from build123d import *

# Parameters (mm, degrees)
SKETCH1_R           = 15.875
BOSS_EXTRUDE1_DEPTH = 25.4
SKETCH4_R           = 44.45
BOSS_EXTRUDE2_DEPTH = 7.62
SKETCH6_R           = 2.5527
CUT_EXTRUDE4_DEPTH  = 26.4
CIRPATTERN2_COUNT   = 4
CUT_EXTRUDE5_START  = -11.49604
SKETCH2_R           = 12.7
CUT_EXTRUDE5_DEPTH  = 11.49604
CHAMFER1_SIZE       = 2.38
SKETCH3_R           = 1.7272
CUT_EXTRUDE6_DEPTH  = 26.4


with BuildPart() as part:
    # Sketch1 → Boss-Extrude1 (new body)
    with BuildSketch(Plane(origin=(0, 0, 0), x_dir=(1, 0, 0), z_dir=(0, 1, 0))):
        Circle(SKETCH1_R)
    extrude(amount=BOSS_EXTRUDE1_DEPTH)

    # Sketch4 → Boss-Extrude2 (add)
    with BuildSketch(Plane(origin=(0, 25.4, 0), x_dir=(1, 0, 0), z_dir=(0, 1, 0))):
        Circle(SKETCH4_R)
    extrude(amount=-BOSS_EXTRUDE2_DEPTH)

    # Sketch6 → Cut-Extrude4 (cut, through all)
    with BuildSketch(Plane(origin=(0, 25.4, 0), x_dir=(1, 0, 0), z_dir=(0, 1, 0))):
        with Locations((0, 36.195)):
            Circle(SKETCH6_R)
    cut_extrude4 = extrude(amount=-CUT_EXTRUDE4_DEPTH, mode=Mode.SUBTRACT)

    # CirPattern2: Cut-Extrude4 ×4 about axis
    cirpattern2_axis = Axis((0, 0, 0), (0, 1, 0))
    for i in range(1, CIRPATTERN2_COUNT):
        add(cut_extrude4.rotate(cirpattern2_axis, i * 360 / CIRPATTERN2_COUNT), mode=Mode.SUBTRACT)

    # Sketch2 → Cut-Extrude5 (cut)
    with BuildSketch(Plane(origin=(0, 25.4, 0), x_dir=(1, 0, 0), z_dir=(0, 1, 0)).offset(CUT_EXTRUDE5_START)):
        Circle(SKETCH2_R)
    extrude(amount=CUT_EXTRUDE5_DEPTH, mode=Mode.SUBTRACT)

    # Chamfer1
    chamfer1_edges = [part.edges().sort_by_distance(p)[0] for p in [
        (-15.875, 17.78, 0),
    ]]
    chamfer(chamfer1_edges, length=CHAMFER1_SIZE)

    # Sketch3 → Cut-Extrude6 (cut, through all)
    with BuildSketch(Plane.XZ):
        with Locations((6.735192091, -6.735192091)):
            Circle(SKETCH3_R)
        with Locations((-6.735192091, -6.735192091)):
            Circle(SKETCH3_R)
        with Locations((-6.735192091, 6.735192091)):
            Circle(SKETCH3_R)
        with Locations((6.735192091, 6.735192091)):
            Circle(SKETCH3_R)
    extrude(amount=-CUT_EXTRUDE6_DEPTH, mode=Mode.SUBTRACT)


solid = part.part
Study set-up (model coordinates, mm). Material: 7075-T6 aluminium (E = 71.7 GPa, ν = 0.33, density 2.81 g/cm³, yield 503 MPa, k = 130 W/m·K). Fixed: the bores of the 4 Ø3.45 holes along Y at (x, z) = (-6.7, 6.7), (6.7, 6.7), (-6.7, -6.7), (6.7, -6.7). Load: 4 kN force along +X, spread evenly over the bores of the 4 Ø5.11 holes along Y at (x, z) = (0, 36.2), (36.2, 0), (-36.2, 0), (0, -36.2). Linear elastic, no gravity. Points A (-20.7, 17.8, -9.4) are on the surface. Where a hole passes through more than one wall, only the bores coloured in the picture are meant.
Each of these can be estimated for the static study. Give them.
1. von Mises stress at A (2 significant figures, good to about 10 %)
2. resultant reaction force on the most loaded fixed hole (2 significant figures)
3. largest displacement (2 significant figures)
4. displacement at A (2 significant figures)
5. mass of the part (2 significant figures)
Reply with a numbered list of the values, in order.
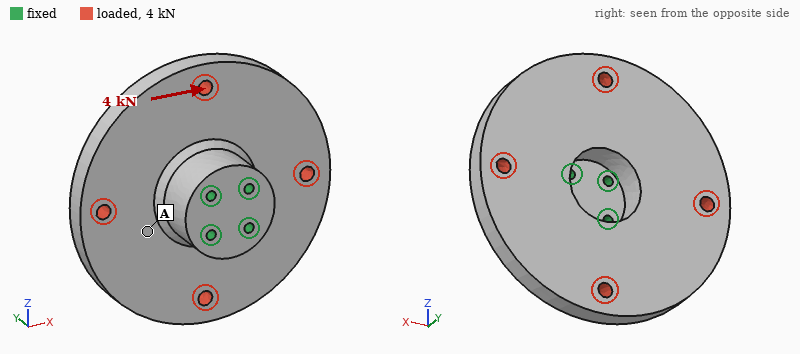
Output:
1. 7.7 MPa
2. 1.5 kN
3. 33 µm
4. 13 µm
5. 150 g
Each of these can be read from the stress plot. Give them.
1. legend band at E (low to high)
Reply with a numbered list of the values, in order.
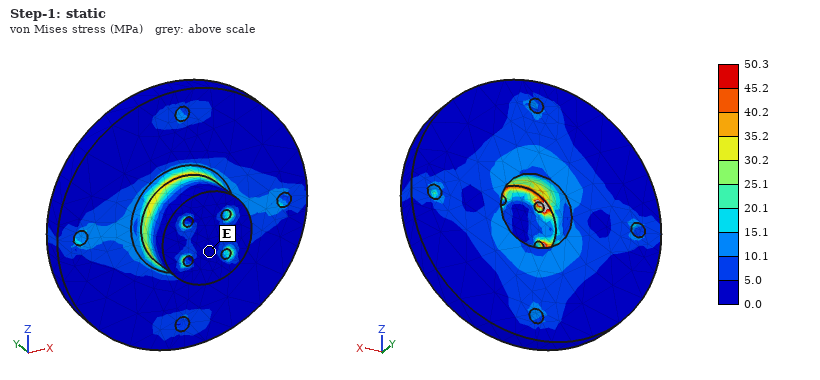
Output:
1. 0.0 to 5.0 MPa
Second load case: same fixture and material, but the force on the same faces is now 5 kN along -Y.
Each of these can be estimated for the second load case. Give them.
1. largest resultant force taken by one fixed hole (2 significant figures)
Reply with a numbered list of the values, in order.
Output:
1. 1.4 kN
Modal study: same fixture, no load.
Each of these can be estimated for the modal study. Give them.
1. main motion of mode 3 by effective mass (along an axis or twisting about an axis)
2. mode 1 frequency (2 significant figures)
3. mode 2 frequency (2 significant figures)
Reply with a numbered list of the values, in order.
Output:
1. along Y
2. 4000 Hz
3. 4000 Hz
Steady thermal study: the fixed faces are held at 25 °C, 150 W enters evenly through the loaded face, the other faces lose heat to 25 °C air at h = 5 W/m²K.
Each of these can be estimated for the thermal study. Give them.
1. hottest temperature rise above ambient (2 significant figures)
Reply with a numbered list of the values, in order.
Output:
1. 66 K
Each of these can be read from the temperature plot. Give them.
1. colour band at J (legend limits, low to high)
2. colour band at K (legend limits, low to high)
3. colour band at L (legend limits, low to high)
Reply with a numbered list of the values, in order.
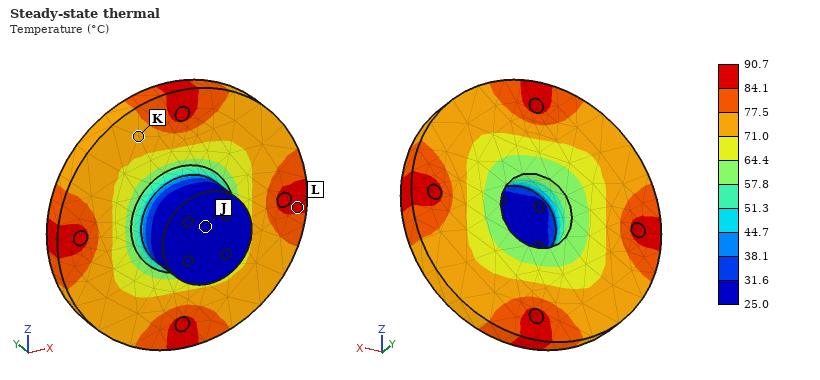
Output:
1. 25.0 to 31.6 °C
2. 71.0 to 77.5 °C
3. 84.1 to 90.7 °C
